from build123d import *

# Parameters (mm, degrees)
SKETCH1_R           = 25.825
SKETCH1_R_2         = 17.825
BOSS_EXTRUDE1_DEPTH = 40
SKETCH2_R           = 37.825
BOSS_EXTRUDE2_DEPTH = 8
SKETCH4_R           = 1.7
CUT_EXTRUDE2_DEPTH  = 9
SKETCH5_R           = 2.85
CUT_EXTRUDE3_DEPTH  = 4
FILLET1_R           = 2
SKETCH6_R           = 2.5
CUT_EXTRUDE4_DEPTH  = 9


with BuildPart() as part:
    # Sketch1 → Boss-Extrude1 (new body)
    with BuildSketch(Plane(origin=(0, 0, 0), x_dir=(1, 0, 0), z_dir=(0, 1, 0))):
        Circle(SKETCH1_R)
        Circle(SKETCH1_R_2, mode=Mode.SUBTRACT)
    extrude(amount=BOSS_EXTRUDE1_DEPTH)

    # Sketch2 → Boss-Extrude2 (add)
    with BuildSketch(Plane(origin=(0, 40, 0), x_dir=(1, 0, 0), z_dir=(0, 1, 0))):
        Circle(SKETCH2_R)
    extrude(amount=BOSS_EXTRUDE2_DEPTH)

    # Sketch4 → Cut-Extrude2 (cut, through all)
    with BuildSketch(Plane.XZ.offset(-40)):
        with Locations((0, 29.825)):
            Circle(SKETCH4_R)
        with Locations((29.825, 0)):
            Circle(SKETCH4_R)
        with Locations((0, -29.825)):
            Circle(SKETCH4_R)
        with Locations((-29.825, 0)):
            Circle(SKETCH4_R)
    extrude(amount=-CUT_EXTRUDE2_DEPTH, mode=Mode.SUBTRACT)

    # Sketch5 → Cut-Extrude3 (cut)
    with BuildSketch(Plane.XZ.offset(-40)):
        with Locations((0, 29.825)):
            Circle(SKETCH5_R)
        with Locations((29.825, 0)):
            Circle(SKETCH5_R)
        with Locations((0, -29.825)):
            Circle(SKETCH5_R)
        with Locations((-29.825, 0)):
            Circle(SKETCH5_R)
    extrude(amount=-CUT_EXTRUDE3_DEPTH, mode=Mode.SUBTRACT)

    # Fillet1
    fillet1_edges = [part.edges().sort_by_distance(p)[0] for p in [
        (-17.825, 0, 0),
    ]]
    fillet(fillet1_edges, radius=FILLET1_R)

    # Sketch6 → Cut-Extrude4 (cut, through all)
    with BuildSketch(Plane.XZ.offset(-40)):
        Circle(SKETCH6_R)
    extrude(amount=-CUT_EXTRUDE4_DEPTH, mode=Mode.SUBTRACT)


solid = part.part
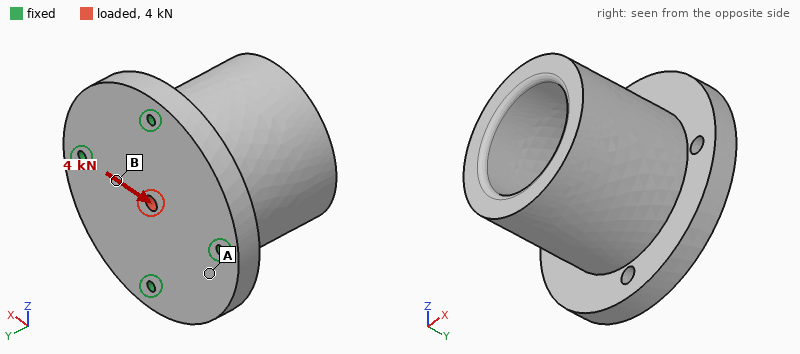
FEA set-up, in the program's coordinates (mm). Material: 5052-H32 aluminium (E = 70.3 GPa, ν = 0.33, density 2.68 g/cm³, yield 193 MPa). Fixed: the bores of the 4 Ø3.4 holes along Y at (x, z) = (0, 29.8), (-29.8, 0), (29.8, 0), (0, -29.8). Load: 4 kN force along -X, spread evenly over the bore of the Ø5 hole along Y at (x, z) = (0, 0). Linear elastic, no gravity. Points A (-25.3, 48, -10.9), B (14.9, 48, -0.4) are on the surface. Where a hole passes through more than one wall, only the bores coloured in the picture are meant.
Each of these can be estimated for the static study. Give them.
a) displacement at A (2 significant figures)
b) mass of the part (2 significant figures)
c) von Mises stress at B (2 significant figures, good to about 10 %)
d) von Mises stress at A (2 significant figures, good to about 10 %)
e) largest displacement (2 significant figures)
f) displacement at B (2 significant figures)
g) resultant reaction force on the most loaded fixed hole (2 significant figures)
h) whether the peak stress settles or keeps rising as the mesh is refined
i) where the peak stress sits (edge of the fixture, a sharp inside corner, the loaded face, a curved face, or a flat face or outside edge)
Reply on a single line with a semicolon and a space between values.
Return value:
2.2 µm; 210 g; 12 MPa; 4.4 MPa; 6.6 µm; 3.3 µm; 1.2 kN; keeps rising; edge of the fixture
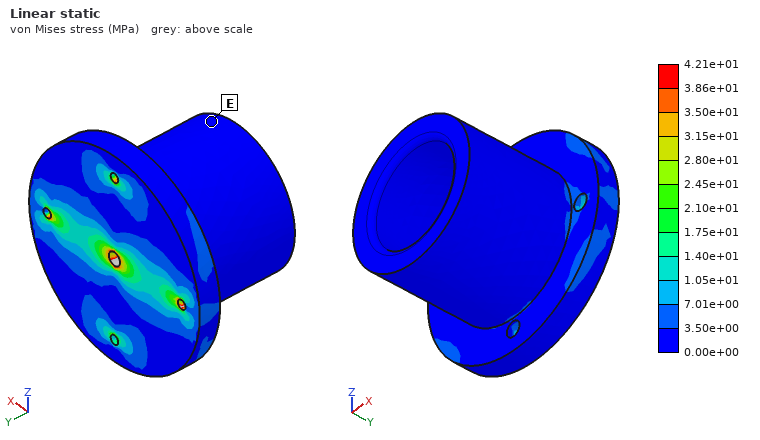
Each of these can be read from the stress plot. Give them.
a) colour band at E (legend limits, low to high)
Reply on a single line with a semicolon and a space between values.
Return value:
0.00e+00 to 3.50e+00 MPa
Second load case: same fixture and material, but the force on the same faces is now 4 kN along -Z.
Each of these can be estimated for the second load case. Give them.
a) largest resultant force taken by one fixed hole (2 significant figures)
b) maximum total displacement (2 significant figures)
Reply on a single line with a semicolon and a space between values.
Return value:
1.2 kN; 6.6 µm
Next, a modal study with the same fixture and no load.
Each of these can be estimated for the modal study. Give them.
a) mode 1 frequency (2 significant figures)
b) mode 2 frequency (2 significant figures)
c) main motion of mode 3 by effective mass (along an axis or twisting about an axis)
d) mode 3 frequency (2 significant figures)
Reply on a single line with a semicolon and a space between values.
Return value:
6800 Hz; 6800 Hz; along Y; 9900 Hz
